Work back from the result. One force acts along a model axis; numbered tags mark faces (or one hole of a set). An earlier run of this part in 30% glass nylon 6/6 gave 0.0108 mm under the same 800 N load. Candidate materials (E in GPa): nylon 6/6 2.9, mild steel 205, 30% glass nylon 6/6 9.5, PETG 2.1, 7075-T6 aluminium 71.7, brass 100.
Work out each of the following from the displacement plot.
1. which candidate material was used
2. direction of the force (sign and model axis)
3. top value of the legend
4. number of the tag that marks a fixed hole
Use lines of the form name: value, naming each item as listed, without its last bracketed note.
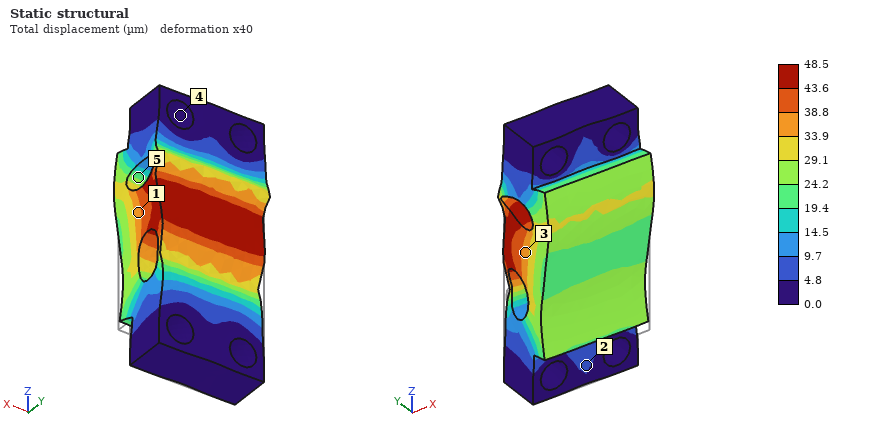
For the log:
which candidate material was used: PETG
direction of the force: +Z
top value of the legend: 48.5 µm
number of the tag that marks a fixed hole: 4
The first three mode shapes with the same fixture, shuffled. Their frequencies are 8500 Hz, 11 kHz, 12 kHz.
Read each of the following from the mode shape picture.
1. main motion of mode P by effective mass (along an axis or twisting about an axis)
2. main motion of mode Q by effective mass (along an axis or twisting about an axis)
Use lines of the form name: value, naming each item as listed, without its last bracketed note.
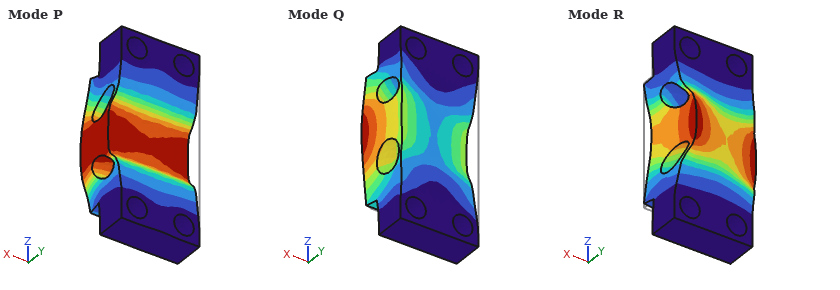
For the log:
main motion of mode P by effective mass: along Y
main motion of mode Q by effective mass: along X
